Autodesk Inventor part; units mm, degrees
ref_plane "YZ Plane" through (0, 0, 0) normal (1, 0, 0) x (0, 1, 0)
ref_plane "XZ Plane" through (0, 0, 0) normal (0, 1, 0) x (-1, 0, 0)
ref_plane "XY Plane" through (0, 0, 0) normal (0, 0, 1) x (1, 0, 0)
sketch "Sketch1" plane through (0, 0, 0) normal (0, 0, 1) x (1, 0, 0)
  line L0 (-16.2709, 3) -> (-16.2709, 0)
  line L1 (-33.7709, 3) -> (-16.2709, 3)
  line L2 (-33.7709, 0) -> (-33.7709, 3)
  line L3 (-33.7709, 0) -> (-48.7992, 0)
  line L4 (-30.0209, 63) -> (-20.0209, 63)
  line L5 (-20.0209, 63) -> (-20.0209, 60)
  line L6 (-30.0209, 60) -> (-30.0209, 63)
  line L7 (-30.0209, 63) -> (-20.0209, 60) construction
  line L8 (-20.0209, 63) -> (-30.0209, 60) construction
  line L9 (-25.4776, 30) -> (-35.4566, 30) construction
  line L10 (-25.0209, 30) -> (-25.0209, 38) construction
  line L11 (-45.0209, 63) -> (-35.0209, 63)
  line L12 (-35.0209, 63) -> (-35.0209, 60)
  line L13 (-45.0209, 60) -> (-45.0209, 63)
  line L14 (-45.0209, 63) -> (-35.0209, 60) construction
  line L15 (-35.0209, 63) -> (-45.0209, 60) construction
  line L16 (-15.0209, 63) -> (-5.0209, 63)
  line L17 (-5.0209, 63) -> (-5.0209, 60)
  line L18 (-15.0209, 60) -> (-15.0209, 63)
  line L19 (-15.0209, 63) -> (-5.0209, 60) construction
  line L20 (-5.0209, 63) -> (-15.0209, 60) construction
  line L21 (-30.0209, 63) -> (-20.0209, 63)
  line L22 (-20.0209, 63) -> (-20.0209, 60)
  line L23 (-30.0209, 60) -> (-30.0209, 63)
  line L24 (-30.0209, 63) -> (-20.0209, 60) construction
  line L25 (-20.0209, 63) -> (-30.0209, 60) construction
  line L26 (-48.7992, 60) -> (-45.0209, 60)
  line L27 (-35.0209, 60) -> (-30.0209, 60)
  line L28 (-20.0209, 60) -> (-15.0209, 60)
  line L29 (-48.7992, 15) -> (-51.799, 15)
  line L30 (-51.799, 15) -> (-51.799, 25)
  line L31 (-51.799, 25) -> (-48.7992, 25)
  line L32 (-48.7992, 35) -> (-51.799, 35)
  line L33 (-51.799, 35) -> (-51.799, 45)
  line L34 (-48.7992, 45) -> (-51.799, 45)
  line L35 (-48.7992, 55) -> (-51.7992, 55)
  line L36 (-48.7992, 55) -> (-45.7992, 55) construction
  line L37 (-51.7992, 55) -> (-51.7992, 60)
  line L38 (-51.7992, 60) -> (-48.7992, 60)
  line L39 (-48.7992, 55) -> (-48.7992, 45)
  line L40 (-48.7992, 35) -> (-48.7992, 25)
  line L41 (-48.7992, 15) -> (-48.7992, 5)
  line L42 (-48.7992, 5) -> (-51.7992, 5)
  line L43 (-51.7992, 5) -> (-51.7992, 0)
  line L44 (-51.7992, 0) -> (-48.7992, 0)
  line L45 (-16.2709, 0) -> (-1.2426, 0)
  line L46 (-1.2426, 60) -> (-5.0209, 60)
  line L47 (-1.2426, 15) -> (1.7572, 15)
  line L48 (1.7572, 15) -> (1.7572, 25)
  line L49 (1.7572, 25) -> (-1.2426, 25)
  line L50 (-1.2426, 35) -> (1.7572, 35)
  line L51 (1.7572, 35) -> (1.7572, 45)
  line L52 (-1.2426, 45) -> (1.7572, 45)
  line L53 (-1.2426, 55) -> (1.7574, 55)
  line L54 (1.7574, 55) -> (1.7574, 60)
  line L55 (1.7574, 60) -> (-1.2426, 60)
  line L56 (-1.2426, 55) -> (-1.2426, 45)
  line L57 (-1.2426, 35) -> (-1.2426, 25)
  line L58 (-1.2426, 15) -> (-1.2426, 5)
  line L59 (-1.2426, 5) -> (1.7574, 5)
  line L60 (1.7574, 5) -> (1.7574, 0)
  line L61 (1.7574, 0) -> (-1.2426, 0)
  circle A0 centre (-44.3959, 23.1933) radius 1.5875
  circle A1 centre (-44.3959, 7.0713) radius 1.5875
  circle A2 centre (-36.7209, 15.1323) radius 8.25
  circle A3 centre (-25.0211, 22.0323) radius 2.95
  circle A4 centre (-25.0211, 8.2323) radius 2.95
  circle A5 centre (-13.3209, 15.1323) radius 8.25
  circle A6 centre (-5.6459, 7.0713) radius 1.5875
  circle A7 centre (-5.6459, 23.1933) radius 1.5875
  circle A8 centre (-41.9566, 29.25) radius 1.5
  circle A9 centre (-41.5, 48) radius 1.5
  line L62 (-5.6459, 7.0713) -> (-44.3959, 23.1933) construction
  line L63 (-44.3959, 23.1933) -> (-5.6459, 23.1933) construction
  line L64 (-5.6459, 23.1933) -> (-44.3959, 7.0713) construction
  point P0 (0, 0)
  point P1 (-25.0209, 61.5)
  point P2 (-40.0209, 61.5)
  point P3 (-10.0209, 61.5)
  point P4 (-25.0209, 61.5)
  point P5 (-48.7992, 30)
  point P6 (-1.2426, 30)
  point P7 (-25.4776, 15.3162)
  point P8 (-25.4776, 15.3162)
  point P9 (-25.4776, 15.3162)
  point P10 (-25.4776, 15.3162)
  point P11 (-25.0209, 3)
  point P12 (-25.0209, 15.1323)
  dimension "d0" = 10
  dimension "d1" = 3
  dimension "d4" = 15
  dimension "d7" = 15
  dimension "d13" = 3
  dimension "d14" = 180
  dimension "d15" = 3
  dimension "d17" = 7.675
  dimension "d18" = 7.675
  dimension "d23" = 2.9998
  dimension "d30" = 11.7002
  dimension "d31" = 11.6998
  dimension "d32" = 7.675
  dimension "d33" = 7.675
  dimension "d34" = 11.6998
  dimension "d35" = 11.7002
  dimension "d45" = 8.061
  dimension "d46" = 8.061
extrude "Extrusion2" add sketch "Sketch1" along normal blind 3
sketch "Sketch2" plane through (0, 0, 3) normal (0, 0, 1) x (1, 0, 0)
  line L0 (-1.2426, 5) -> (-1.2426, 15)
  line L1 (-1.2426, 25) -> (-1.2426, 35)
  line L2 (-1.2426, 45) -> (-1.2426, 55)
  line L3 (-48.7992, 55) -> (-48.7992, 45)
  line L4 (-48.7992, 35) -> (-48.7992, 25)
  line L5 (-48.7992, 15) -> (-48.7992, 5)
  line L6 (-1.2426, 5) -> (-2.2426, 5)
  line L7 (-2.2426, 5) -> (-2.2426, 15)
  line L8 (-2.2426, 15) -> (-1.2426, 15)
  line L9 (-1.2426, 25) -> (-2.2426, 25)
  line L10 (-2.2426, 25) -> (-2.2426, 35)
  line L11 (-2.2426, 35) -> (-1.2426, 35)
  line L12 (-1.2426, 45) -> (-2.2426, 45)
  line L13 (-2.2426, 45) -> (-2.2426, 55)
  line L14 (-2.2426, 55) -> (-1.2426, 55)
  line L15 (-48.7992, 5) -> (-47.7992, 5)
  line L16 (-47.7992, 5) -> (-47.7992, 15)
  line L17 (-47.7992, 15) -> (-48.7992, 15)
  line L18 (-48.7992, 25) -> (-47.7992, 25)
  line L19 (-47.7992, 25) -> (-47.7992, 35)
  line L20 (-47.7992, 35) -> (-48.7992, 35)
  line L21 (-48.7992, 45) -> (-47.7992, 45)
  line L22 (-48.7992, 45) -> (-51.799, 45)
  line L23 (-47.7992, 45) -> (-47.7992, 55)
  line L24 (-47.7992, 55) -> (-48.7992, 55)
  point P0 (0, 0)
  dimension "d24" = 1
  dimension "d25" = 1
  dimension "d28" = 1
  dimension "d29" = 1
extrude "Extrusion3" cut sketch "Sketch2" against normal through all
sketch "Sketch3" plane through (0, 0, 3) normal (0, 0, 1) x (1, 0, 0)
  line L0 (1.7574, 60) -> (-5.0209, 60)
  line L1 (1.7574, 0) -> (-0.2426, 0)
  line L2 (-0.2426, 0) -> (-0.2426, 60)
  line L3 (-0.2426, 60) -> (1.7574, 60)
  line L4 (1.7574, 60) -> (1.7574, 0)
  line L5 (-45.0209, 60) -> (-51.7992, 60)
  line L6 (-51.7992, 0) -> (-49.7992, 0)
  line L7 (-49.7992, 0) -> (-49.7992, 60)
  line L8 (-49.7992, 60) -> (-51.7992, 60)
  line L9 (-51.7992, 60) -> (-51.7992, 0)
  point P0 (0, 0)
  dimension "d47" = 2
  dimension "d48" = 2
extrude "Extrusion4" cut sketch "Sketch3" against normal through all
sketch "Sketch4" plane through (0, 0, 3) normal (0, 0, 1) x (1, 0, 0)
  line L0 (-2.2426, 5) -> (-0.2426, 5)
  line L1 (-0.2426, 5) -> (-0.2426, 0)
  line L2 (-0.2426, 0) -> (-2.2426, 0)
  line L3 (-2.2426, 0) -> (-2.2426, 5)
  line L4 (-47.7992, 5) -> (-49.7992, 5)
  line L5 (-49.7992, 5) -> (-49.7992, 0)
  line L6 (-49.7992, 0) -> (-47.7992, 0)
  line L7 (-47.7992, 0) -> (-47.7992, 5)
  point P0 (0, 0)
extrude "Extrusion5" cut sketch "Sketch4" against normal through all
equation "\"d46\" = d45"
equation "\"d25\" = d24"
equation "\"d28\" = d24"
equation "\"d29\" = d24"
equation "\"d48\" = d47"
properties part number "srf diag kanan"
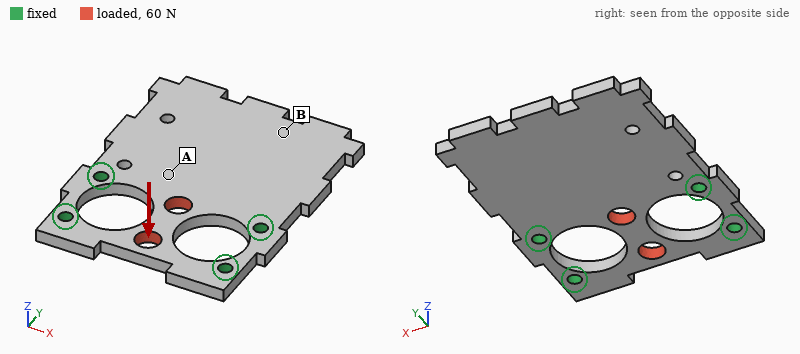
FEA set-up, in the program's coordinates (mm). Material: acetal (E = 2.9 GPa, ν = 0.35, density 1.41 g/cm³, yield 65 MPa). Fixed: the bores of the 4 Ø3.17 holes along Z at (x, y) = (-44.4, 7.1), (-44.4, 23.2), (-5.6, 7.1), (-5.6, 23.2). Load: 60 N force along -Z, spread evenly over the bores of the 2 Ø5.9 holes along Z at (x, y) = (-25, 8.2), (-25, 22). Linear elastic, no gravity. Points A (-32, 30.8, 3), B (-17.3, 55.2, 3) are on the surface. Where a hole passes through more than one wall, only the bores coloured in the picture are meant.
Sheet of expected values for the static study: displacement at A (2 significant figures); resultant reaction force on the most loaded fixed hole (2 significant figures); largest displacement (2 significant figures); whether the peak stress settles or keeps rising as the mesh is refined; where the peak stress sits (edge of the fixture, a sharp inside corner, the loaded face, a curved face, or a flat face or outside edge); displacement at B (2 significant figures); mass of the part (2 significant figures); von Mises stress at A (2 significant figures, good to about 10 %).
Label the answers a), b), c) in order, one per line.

a) 0.060 mm
b) 16 N
c) 0.24 mm
d) keeps rising
e) edge of the fixture
f) 0.073 mm
g) 9.9 g
h) 3.7 MPa
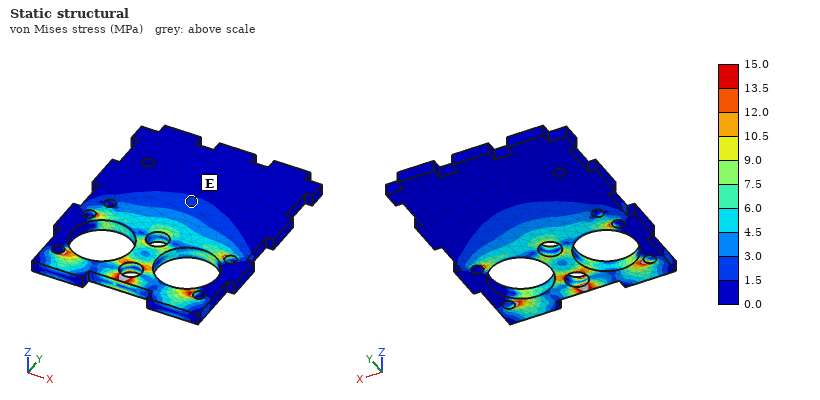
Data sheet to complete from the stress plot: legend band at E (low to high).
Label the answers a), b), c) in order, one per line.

a) 1.5 to 3.0 MPa
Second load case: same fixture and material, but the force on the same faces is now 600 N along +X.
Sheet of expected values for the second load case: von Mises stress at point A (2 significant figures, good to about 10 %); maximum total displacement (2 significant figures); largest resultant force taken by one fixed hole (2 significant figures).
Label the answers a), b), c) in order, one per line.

a) 2.6 MPa
b) 0.13 mm
c) 170 N
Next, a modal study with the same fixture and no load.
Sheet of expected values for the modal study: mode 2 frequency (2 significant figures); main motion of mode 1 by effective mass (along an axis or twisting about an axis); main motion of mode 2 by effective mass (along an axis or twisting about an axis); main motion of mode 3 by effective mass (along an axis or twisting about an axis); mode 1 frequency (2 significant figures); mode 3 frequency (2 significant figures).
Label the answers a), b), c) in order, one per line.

a) 940 Hz
b) along Z
c) twisting about Y
d) along Z
e) 370 Hz
f) 2200 Hz
